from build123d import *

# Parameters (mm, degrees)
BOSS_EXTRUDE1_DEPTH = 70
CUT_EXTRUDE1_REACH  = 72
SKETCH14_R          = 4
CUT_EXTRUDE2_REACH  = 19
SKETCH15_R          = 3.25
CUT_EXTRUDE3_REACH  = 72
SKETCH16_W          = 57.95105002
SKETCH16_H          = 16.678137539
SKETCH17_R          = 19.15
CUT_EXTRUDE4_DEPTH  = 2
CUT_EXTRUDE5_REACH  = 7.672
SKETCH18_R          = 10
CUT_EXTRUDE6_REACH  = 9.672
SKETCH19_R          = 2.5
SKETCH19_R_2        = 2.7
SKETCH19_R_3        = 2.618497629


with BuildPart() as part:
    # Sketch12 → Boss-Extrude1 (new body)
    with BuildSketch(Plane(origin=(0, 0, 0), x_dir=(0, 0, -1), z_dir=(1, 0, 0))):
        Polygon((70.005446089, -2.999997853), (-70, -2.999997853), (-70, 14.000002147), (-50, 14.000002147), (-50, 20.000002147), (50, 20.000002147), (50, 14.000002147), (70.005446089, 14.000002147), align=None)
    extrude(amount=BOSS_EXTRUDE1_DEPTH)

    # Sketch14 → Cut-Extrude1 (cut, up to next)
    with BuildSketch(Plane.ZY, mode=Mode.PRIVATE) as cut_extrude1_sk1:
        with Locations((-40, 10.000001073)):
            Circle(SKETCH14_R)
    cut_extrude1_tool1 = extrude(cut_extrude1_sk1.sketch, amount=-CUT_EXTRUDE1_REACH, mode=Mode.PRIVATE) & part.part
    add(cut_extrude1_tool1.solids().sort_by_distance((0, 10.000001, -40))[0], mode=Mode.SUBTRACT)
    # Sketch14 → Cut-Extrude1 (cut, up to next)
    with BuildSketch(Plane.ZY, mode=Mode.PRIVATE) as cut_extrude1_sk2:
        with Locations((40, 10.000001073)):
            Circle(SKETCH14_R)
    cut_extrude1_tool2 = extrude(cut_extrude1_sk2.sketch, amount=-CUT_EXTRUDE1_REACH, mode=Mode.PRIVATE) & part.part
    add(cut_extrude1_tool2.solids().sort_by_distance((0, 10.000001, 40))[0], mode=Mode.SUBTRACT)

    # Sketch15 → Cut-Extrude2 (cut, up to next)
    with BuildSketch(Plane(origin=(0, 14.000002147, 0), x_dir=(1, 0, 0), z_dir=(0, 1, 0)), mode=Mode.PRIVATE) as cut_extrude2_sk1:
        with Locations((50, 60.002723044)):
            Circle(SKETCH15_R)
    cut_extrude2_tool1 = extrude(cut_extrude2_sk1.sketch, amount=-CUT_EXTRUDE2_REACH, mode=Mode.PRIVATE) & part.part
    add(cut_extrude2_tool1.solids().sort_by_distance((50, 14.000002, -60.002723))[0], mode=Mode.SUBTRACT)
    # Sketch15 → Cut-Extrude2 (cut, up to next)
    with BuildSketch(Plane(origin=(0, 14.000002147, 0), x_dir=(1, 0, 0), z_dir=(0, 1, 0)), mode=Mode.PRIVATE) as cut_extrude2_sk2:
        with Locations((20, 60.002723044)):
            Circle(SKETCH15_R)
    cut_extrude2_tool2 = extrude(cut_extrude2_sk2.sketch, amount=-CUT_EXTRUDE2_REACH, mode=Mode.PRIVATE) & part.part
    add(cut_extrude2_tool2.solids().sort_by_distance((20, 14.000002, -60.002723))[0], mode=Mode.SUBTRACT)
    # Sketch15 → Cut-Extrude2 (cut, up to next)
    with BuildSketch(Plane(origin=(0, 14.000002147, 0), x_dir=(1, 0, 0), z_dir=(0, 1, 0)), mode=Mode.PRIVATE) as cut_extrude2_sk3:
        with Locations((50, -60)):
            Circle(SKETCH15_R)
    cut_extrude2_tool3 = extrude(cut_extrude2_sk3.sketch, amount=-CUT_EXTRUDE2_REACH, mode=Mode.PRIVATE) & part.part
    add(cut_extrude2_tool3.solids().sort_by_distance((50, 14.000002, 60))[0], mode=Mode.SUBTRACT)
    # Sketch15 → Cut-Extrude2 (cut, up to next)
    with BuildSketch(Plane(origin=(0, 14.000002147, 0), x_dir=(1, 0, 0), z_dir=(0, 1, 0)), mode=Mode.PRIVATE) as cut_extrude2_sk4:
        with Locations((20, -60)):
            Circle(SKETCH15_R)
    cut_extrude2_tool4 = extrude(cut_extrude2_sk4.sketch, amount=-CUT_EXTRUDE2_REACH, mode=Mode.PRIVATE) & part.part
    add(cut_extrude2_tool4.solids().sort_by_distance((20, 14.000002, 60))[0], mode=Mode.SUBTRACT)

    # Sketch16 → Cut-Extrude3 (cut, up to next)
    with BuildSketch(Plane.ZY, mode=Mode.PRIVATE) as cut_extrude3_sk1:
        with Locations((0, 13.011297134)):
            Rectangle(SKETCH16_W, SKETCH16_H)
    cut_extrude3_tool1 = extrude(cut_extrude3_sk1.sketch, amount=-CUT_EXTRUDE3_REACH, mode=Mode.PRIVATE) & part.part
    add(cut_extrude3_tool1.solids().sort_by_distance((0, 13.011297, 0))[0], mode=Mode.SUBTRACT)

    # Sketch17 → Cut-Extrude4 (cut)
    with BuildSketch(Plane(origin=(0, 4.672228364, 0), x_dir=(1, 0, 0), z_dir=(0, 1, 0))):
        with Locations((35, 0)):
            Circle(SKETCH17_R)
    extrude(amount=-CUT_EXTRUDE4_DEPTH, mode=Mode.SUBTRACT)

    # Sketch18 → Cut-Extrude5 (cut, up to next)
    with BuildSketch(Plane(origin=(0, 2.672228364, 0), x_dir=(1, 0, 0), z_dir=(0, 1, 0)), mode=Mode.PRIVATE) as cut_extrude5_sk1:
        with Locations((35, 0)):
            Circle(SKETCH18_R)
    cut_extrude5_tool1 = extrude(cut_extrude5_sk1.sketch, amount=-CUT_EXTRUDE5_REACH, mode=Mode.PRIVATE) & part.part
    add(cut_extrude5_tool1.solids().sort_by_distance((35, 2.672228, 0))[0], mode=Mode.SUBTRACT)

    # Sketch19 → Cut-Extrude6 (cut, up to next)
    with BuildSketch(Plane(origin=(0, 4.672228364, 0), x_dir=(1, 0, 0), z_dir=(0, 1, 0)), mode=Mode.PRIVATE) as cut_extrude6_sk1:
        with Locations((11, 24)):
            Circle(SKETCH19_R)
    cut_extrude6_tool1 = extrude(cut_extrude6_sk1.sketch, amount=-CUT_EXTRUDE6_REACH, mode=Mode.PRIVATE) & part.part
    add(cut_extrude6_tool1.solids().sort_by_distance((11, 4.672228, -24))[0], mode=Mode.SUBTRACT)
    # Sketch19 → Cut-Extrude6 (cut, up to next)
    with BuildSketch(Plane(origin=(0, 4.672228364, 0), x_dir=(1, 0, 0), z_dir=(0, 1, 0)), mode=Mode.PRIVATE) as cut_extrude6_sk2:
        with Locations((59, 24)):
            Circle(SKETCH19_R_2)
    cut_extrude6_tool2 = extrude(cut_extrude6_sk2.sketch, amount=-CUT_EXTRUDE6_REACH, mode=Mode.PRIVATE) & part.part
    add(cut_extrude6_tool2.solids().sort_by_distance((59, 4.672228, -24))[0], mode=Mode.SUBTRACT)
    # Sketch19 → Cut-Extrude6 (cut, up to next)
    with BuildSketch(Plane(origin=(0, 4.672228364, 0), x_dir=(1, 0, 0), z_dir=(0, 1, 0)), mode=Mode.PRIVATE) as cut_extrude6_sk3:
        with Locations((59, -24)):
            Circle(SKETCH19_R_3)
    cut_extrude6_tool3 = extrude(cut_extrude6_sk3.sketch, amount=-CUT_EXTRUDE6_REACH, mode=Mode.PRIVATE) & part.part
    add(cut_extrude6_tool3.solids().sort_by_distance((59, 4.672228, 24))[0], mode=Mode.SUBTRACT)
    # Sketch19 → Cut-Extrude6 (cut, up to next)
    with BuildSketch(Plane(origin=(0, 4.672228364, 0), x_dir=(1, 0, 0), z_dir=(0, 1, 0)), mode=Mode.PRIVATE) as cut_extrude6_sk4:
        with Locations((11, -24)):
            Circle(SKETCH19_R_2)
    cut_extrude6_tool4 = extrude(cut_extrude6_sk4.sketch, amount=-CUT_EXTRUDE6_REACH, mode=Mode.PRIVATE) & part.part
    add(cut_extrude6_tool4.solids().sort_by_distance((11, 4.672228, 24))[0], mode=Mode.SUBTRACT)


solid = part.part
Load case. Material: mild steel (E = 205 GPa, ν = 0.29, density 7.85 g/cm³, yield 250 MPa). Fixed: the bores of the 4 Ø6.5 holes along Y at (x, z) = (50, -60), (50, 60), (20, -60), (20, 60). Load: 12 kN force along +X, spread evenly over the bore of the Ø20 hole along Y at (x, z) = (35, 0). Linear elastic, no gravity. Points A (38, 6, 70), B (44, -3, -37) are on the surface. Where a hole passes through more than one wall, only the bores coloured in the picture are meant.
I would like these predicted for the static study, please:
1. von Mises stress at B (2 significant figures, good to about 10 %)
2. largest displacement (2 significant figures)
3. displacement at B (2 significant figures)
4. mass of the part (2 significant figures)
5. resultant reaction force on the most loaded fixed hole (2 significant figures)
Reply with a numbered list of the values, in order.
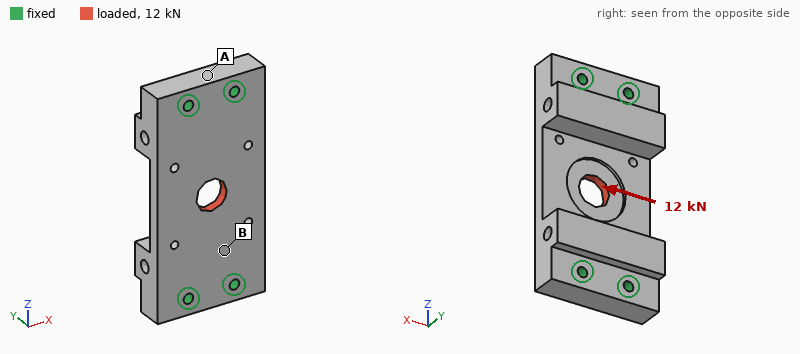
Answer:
1. 25 MPa
2. 13 µm
3. 4.2 µm
4. 1.0 kg
5. 5.6 kN
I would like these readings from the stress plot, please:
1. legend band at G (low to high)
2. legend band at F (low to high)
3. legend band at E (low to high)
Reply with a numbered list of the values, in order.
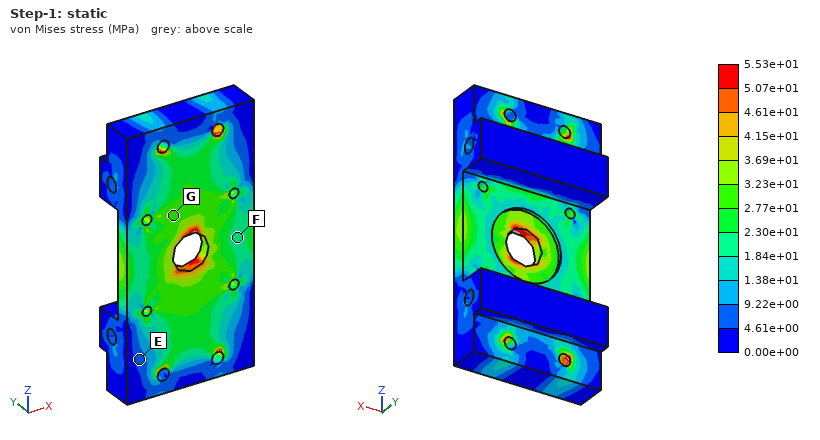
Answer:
1. 2.77e+01 to 3.23e+01 MPa
2. 1.84e+01 to 2.30e+01 MPa
3. 4.61e+00 to 9.22e+00 MPa
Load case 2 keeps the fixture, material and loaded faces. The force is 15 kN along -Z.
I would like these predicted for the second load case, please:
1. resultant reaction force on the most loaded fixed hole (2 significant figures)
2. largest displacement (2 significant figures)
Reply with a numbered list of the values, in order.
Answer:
1. 3.8 kN
2. 6.7 µm
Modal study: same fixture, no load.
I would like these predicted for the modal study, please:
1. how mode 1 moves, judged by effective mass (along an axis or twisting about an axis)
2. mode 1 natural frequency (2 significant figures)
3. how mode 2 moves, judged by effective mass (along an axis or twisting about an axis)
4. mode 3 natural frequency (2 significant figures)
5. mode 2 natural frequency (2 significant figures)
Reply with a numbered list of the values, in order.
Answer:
1. along Y
2. 5300 Hz
3. twisting about Z
4. 8300 Hz
5. 7100 Hz
